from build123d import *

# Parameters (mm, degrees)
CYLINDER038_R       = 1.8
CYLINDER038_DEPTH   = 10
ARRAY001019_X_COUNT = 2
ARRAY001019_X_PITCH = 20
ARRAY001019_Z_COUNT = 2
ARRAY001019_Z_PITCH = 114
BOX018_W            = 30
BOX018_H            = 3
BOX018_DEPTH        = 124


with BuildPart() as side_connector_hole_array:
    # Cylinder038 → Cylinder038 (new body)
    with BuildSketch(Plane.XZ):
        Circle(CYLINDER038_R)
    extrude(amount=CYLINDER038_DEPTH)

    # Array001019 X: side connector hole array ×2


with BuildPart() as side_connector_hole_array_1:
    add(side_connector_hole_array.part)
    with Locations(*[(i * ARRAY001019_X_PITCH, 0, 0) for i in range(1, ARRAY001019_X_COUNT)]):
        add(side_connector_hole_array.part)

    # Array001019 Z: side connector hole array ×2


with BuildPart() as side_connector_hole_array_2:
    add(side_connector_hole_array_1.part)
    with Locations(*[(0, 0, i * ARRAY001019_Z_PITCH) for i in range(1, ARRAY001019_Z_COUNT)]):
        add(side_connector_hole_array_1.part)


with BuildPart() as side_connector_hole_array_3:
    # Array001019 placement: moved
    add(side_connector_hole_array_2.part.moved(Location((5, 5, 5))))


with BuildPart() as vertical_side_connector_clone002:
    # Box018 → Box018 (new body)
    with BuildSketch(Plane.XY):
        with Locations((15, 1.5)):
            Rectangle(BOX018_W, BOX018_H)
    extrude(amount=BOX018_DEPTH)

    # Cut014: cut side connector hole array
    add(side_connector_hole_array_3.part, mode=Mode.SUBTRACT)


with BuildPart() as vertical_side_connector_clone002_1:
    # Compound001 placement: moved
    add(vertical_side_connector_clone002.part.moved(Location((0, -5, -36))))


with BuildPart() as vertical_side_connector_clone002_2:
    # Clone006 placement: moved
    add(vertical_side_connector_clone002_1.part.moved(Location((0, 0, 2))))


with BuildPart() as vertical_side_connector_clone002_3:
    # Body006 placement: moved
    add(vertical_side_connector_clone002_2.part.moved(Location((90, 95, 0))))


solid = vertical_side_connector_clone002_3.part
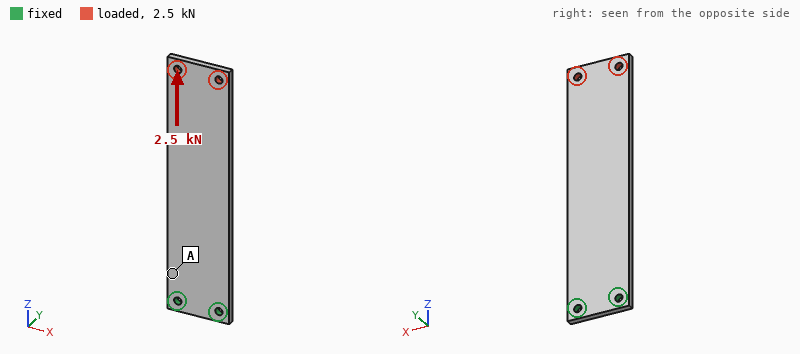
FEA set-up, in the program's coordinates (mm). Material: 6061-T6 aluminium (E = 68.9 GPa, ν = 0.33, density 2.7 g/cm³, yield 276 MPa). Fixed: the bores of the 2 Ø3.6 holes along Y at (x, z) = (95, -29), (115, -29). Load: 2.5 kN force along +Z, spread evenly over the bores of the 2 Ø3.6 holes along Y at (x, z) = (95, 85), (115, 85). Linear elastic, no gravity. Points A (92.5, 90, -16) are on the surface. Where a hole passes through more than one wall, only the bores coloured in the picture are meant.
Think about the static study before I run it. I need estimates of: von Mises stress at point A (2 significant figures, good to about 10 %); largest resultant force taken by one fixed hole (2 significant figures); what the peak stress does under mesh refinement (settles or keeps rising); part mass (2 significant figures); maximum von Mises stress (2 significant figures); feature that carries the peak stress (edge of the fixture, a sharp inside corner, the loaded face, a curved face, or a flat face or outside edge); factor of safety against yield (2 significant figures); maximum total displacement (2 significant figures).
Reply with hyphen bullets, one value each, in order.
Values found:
- 30 MPa
- 1.3 kN
- settles
- 30 g
- 100 MPa
- the loaded face
- 2.8
- 52 µm
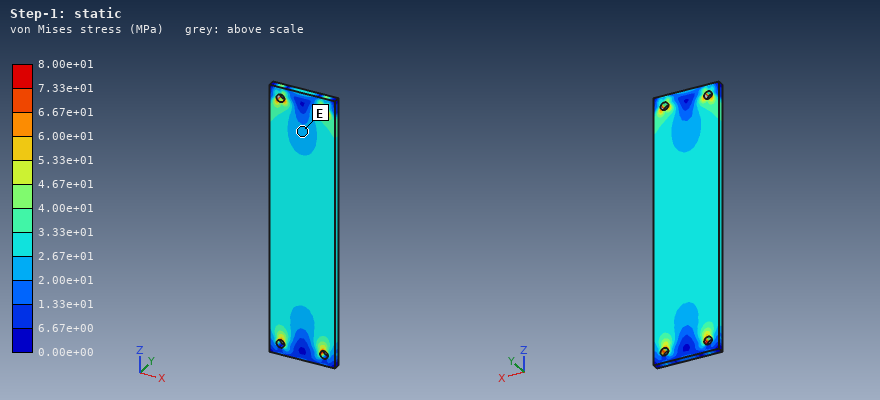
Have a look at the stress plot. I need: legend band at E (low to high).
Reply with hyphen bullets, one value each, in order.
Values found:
- 2.00e+01 to 2.67e+01 MPa
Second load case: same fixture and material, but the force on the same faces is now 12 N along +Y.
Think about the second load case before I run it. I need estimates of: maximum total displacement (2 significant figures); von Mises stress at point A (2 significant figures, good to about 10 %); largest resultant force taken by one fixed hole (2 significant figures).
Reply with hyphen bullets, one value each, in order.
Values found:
- 1.3 mm
- 27 MPa
- 6.0 N
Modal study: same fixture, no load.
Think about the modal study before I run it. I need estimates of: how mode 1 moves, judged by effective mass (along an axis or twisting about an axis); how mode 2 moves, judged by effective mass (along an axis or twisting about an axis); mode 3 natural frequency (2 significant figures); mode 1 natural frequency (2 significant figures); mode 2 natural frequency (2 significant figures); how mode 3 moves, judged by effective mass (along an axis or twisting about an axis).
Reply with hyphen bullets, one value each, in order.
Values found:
- along Y
- along Y
- 1400 Hz
- 180 Hz
- 1100 Hz
- twisting about Z
